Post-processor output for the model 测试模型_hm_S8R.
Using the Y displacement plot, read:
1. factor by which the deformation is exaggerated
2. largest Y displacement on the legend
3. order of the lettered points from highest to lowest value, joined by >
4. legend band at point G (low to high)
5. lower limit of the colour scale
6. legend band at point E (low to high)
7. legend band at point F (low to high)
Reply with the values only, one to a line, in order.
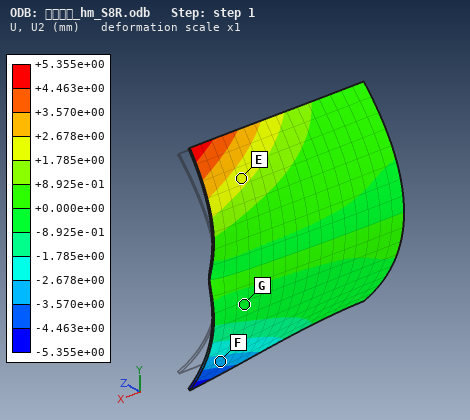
1
+5.355e+00 mm
E > G > F
-8.925e-01 to +0.000e+00 mm
-5.355e+00 mm
+1.785e+00 to +2.678e+00 mm
-3.570e+00 to -2.678e+00 mm
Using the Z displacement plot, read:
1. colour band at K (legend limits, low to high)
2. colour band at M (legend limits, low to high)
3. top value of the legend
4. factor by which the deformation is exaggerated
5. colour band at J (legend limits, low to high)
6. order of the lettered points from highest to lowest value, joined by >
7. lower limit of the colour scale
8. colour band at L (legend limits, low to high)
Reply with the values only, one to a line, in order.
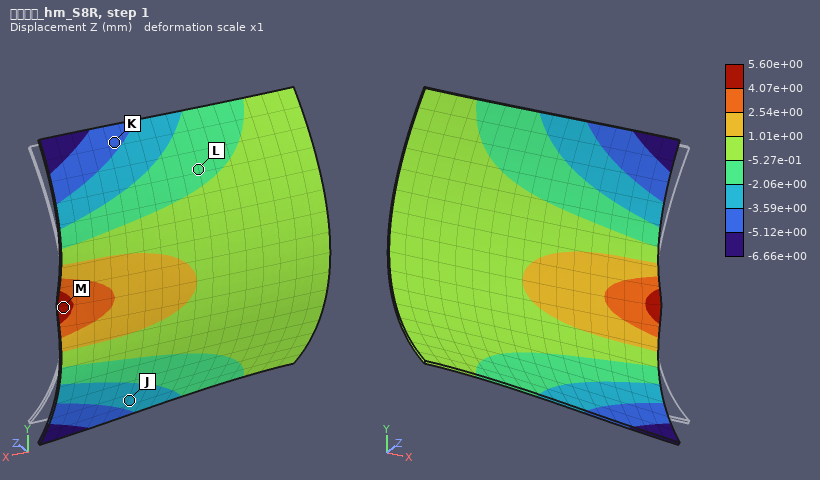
-5.12e+00 to -3.59e+00 mm
4.07e+00 to 5.60e+00 mm
5.60e+00 mm
1
-3.59e+00 to -2.06e+00 mm
M > L > J > K
-6.66e+00 mm
-2.06e+00 to -5.27e-01 mm
